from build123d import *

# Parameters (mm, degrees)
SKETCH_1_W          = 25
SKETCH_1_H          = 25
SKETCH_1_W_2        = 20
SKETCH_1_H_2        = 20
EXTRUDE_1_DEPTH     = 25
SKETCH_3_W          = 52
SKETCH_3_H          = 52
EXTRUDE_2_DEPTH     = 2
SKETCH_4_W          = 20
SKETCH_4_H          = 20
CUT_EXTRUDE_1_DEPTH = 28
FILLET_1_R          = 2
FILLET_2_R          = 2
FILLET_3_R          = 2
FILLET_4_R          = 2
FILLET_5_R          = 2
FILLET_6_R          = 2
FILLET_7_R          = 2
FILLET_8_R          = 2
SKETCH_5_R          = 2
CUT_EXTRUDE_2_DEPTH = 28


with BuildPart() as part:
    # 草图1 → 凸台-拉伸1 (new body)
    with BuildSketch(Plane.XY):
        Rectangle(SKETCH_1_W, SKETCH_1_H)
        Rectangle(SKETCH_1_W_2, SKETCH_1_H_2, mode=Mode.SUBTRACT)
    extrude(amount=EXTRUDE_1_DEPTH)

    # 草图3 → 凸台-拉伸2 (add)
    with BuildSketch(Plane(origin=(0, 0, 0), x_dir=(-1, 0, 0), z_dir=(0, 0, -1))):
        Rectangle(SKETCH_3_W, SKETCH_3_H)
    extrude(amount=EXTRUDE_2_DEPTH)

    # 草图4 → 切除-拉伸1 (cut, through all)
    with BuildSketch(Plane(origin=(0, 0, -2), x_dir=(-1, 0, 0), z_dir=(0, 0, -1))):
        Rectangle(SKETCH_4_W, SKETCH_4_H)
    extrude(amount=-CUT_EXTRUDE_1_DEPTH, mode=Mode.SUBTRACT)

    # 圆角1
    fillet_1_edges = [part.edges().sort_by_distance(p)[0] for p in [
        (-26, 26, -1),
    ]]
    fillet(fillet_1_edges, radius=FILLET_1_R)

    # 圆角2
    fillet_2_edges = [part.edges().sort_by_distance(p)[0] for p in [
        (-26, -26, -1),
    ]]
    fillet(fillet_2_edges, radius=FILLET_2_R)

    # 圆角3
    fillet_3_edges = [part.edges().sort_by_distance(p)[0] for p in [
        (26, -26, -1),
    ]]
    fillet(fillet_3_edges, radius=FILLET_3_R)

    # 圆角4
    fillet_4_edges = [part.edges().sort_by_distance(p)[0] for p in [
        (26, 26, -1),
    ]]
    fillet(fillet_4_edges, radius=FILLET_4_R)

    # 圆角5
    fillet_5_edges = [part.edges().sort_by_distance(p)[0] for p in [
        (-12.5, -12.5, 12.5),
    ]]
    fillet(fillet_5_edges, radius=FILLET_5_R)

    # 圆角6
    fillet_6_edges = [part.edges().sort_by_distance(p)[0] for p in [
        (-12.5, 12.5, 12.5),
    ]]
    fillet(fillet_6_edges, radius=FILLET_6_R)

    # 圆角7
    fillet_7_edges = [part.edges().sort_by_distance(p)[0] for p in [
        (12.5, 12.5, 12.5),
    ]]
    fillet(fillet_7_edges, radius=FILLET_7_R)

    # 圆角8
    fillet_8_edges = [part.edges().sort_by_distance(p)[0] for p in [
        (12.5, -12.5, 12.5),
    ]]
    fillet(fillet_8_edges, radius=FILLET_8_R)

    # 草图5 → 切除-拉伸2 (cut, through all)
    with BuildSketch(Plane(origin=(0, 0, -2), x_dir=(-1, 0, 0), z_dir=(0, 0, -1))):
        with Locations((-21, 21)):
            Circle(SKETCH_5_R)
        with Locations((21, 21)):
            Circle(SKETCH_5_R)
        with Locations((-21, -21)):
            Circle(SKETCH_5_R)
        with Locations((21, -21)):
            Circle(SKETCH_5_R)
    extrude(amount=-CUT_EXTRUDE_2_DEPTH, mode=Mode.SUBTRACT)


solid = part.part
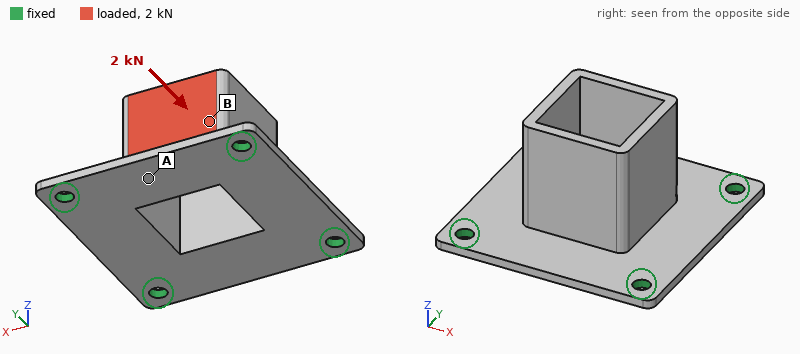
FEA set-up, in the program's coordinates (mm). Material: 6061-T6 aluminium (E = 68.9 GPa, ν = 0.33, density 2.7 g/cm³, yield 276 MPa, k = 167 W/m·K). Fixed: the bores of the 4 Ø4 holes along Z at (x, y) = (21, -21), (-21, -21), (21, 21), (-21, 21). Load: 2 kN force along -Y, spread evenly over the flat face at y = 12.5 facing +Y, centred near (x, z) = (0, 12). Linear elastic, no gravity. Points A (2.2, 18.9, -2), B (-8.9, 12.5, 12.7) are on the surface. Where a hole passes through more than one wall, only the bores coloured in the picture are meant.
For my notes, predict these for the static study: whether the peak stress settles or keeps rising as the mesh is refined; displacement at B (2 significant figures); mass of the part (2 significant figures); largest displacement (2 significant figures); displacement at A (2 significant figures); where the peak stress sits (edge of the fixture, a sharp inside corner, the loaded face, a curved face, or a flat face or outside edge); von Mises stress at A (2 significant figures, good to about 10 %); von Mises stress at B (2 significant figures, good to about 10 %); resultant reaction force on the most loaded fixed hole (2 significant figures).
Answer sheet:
keeps rising
0.16 mm
27 g
0.30 mm
0.12 mm
edge of the fixture
68 MPa
29 MPa
700 N
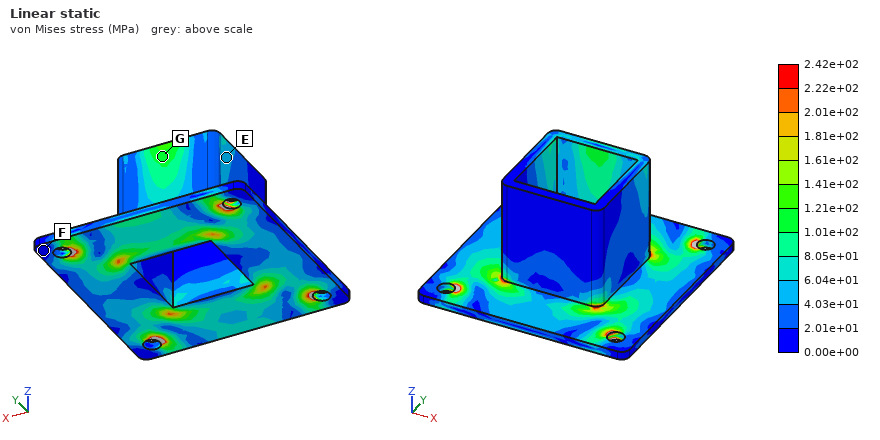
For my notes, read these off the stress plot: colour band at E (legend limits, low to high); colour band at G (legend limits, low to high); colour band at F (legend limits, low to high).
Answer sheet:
4.03e+01 to 6.04e+01 MPa
1.01e+02 to 1.21e+02 MPa
0.00e+00 to 2.01e+01 MPa
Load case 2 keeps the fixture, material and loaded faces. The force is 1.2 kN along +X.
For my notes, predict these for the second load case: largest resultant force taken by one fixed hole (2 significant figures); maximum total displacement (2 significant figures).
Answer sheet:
550 N
0.17 mm
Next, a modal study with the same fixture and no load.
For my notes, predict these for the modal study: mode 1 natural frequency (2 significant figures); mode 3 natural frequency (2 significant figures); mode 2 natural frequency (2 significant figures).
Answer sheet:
3900 Hz
3900 Hz
3900 Hz
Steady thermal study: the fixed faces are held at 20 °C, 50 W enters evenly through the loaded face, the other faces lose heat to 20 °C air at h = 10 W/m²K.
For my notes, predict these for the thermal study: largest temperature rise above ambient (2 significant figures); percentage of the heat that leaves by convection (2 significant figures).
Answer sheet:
67 K
5.0 %
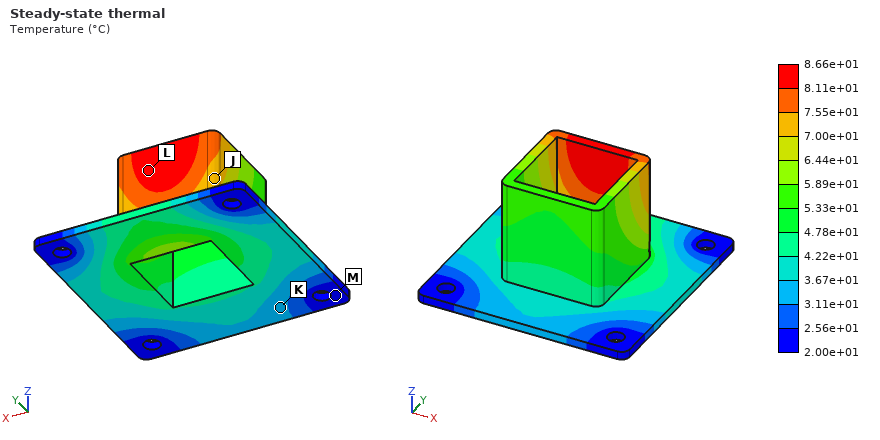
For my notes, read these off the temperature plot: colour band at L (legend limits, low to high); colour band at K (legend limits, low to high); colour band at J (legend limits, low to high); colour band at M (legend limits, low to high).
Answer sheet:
8.11e+01 to 8.66e+01 °C
3.11e+01 to 3.67e+01 °C
7.00e+01 to 7.55e+01 °C
2.00e+01 to 2.56e+01 °C
